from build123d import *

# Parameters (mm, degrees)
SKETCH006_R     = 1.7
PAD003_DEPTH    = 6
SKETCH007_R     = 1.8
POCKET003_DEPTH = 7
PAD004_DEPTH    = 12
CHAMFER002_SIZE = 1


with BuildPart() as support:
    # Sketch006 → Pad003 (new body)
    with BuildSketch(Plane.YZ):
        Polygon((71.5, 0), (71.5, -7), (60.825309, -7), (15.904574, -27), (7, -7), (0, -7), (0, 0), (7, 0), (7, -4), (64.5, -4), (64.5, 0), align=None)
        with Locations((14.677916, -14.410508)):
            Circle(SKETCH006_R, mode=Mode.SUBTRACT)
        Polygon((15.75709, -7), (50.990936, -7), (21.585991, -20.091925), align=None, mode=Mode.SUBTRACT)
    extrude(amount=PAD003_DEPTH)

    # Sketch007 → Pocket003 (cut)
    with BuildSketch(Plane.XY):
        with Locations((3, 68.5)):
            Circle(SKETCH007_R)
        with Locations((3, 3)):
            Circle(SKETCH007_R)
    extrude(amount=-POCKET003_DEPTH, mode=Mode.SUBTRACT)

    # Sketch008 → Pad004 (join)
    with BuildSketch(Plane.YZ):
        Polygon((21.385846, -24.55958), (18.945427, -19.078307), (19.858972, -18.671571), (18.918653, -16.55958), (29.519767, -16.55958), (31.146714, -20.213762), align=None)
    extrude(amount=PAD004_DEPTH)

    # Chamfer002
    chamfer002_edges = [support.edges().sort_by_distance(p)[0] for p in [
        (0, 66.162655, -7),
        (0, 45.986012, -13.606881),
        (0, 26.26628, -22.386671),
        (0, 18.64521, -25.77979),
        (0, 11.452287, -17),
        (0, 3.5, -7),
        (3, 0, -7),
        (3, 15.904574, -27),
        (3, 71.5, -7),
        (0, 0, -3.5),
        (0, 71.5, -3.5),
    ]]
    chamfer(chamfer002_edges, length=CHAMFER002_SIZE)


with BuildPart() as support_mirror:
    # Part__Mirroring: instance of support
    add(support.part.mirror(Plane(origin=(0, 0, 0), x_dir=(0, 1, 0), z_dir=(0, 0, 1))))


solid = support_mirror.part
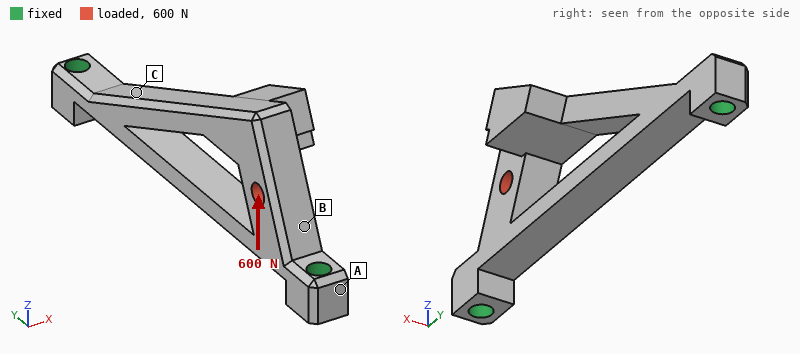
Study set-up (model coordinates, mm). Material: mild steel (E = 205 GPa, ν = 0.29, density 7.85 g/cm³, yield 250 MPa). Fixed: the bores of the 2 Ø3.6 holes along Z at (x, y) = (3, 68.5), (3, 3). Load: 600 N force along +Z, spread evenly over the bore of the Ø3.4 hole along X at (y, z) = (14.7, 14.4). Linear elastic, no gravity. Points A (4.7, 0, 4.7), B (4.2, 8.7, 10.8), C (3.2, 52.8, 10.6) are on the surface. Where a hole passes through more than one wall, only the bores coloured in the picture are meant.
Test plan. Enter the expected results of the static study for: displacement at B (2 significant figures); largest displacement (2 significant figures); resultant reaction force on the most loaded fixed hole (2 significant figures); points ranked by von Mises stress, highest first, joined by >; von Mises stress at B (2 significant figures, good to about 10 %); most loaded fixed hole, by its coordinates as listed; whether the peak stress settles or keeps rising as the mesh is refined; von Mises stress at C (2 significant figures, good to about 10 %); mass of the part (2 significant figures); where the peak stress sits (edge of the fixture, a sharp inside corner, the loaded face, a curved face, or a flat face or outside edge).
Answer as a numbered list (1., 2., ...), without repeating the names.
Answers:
1. 3.2 µm
2. 6.2 µm
3. 550 N
4. B > C > A
5. 42 MPa
6. (3, 3)
7. keeps rising
8. 17 MPa
9. 29 g
10. edge of the fixture
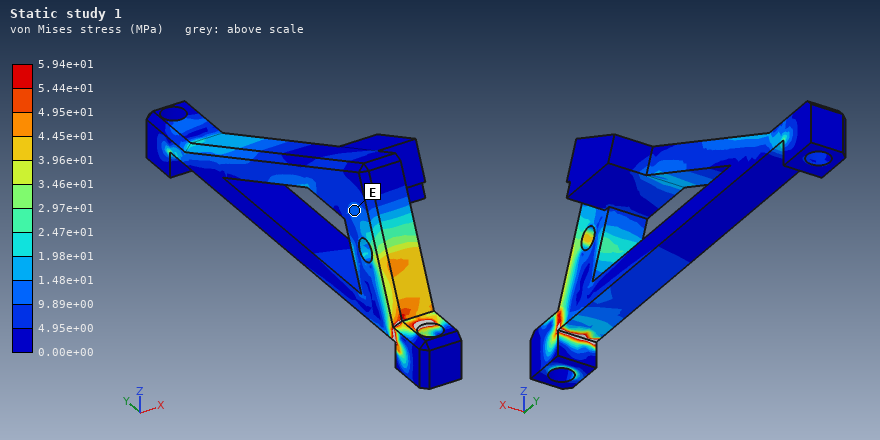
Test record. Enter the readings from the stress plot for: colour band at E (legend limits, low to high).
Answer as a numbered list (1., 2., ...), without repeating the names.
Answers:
1. 9.89e+00 to 1.48e+01 MPa
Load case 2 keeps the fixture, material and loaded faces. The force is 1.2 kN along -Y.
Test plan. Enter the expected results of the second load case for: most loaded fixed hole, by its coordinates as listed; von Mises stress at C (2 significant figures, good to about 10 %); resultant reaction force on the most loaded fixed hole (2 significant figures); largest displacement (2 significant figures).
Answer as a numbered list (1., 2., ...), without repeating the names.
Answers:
1. (3, 3)
2. 42 MPa
3. 730 N
4. 8.1 µm
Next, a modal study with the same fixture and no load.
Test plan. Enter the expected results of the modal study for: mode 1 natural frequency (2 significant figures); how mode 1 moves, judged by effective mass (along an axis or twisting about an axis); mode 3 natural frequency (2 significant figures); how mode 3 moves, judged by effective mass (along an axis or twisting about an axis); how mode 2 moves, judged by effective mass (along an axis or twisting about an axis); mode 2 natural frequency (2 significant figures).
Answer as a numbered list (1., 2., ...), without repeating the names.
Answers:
1. 3200 Hz
2. along X
3. 7300 Hz
4. along X
5. along Z
6. 6100 Hz
